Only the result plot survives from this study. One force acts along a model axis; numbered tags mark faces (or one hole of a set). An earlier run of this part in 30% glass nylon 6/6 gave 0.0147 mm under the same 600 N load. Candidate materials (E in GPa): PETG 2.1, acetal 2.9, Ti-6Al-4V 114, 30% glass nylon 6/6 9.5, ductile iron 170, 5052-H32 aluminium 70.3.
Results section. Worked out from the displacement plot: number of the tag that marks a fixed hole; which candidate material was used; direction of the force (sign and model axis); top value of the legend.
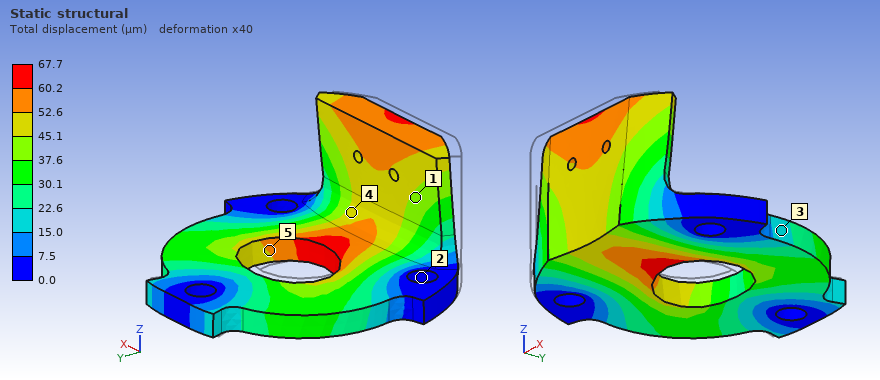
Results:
2
PETG
+Y
67.7 µm
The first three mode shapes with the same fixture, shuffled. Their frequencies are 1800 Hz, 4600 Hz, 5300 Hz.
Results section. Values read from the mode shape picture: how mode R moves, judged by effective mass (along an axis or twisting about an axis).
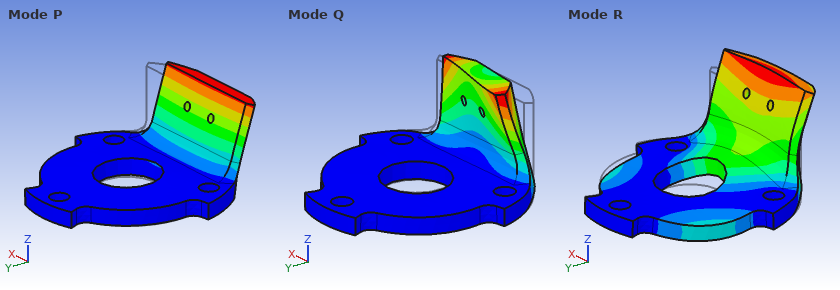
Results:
along Z
